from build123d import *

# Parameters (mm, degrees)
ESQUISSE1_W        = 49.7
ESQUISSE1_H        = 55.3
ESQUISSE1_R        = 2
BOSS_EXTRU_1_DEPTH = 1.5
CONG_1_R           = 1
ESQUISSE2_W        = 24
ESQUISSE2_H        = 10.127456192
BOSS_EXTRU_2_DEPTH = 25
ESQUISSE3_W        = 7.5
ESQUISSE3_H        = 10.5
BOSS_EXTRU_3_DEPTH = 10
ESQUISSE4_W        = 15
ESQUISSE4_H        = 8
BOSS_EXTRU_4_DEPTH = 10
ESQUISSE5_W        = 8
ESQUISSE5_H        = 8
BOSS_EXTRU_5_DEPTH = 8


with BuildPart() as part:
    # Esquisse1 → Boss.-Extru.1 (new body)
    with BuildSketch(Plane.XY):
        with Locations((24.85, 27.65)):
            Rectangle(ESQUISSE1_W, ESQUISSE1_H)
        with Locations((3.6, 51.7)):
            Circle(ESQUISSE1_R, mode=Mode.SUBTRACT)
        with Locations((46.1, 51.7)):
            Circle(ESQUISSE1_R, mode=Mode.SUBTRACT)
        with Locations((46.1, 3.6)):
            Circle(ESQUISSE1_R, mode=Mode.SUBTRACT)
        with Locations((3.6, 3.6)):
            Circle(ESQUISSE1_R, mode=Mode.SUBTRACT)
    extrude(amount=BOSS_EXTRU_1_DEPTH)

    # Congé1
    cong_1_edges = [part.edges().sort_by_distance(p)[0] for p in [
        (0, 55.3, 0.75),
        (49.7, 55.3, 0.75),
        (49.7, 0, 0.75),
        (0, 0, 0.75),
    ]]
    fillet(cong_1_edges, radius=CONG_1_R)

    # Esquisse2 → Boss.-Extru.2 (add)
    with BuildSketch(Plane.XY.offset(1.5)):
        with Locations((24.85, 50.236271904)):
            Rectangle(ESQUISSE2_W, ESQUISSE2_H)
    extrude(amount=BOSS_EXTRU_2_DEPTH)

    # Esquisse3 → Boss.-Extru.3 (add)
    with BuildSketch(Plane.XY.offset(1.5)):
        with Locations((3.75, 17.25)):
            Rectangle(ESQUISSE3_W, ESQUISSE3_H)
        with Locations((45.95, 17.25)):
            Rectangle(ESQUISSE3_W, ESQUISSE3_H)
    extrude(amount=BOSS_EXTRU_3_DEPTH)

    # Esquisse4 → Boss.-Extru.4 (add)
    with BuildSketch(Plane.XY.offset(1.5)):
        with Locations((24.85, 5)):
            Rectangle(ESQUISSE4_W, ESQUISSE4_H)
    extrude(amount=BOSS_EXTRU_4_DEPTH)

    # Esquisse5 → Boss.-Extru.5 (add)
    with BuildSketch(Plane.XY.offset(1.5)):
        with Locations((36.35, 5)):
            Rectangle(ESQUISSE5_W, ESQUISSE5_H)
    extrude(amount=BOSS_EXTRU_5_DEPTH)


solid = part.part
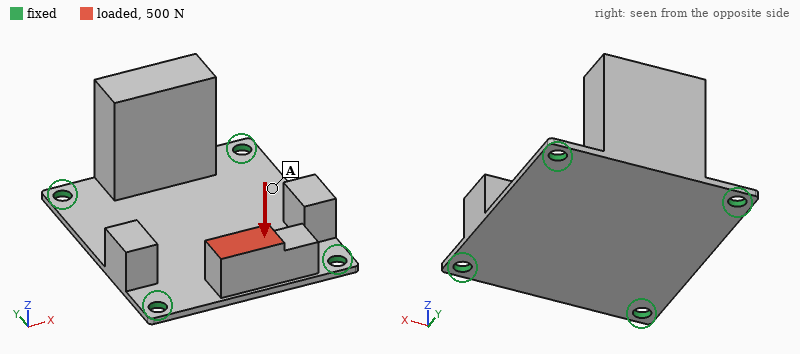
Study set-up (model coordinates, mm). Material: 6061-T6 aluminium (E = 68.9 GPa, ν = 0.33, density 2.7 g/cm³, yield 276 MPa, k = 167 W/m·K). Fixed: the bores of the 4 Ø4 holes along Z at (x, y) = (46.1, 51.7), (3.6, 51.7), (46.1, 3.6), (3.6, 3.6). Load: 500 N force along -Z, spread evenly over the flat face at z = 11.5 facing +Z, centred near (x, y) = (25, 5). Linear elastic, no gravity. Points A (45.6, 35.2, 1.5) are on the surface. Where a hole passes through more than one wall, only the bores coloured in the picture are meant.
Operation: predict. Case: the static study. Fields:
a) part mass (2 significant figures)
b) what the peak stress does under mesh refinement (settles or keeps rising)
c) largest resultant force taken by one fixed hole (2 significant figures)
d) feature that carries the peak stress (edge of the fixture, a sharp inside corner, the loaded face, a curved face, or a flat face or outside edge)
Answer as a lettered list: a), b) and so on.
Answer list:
a) 36 g
b) keeps rising
c) 290 N
d) edge of the fixture
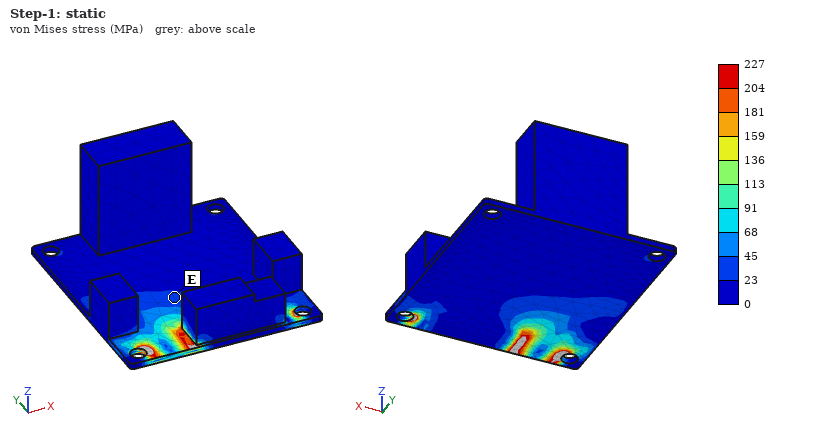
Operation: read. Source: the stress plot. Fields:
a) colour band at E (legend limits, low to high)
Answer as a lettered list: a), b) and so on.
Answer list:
a) 23 to 45 MPa
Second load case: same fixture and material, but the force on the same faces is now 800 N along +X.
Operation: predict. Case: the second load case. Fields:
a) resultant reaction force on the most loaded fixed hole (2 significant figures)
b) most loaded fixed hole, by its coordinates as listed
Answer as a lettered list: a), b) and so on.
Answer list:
a) 510 N
b) (46.1, 3.6)
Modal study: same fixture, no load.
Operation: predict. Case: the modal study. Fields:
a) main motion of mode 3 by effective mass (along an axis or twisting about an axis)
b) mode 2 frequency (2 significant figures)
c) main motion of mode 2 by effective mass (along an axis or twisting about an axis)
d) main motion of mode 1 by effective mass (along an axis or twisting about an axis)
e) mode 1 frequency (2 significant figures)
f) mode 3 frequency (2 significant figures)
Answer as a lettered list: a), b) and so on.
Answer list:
a) along X
b) 2800 Hz
c) along Z
d) along Y
e) 1100 Hz
f) 3100 Hz
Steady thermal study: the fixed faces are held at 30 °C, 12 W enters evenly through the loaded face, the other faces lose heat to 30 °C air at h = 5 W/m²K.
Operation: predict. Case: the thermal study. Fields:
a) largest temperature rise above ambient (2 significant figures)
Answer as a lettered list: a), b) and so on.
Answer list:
a) 22 K
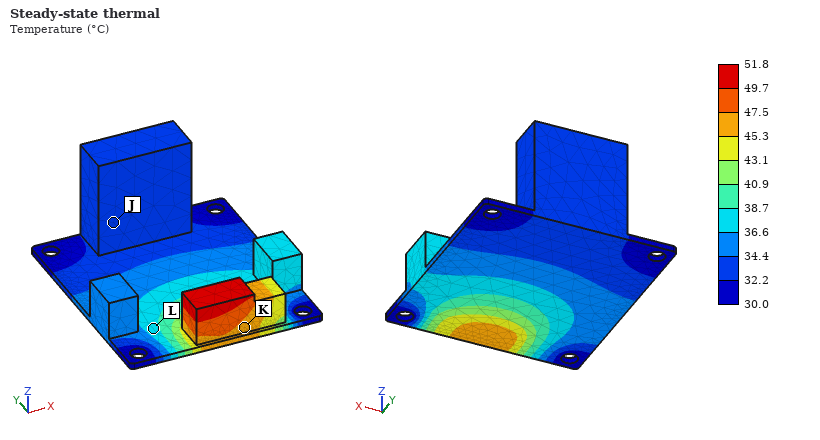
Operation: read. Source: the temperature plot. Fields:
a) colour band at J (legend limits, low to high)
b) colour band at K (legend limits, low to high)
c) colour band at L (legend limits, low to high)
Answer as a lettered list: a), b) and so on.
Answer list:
a) 32.2 to 34.4 °C
b) 45.3 to 47.5 °C
c) 36.6 to 38.7 °C
